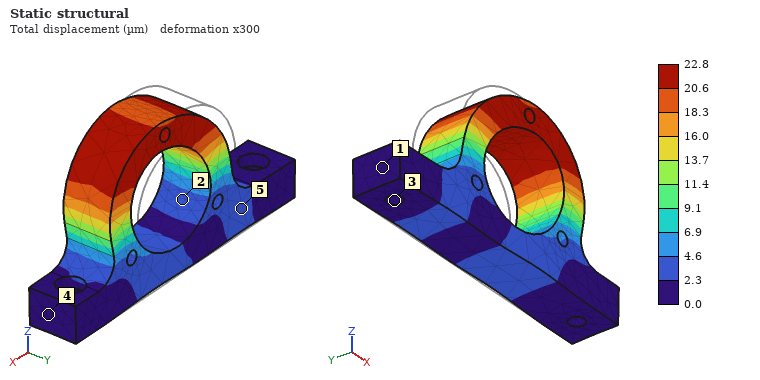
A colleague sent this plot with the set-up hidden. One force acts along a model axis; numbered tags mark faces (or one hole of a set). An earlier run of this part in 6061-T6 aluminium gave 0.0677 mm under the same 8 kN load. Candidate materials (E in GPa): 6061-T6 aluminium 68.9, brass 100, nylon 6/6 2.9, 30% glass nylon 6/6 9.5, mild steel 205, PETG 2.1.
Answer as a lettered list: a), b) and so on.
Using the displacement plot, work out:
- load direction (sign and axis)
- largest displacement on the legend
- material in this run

a) +X
b) 22.8 µm
c) mild steel
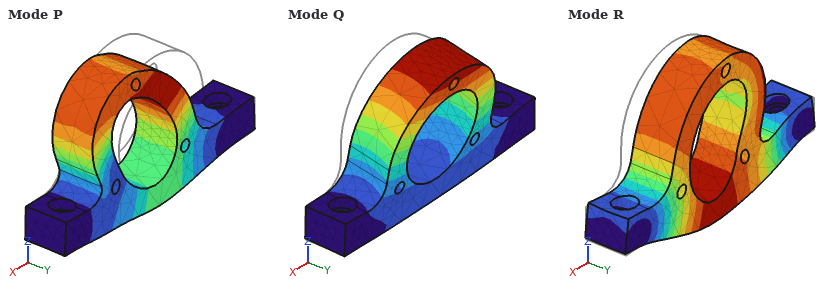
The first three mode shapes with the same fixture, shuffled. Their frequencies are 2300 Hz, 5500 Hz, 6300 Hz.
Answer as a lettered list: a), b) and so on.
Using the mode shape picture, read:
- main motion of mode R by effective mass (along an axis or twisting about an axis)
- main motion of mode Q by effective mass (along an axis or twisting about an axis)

a) along Z
b) along Y
